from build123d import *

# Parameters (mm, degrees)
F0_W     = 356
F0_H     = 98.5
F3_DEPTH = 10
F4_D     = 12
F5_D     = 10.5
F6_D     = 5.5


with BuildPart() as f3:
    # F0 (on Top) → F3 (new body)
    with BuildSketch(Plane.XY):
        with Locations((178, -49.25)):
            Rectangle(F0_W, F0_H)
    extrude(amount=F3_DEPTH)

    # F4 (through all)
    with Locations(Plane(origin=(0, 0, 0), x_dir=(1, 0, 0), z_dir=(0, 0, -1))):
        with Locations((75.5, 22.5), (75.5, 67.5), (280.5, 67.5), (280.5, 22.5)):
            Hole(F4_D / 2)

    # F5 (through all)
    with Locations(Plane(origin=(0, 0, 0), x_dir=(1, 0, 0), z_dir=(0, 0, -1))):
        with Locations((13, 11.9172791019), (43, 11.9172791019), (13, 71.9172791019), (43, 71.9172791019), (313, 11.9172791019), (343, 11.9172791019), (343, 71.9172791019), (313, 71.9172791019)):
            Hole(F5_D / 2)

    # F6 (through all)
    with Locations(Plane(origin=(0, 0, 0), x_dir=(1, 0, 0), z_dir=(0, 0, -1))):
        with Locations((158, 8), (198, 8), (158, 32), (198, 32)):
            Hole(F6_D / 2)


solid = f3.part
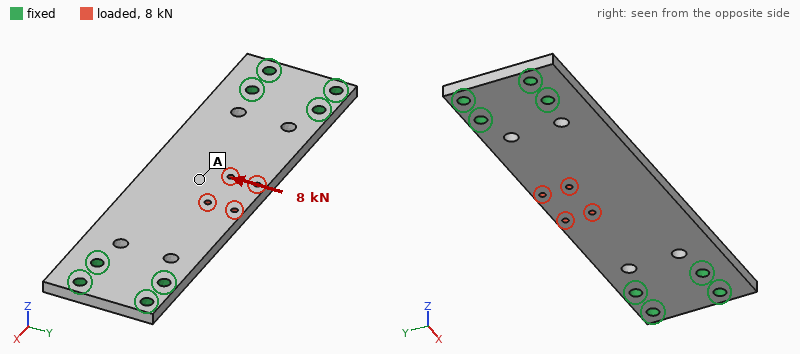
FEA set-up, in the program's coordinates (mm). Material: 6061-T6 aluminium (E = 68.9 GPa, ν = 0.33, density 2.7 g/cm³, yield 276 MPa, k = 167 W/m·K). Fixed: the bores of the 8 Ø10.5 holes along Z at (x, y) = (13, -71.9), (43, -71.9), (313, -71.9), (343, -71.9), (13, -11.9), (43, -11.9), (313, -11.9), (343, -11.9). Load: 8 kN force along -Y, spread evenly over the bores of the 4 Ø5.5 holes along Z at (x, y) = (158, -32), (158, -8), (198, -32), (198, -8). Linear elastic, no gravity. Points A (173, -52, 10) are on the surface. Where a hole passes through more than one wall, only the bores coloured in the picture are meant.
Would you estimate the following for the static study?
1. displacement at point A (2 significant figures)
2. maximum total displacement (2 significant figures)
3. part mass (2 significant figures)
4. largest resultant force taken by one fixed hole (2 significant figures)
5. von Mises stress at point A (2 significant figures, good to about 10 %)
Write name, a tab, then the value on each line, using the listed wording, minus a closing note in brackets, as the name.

displacement at point A	40 µm
maximum total displacement	42 µm
part mass	910 g
largest resultant force taken by one fixed hole	3.7 kN
von Mises stress at point A	4.8 MPa
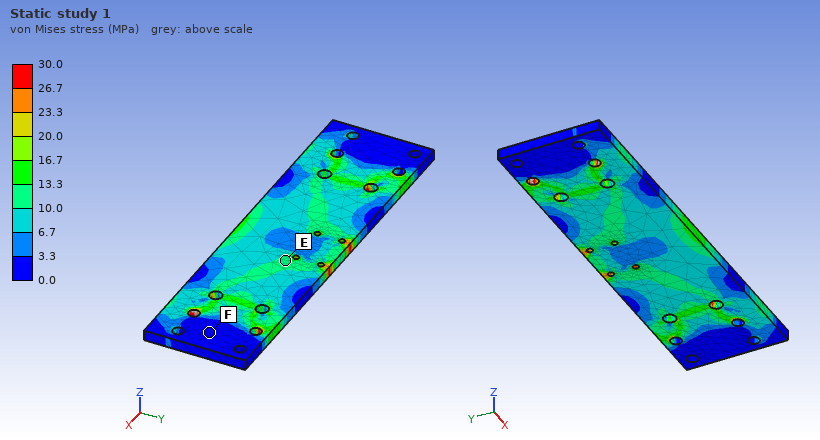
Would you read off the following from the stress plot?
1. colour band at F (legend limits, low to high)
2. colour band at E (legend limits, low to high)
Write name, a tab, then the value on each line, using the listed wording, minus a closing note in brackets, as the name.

colour band at F	0.0 to 3.3 MPa
colour band at E	10.0 to 13.3 MPa
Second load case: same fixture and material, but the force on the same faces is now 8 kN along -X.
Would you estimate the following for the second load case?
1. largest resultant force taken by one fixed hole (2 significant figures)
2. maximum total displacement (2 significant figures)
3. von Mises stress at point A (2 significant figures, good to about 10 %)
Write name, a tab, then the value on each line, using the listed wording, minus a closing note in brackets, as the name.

largest resultant force taken by one fixed hole	1.9 kN
maximum total displacement	13 µm
von Mises stress at point A	2.8 MPa
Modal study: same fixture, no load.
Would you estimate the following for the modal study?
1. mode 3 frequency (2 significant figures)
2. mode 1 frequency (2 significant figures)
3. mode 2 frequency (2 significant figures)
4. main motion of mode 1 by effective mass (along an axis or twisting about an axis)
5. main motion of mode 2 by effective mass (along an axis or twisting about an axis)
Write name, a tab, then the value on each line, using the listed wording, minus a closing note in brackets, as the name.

mode 3 frequency	2000 Hz
mode 1 frequency	710 Hz
mode 2 frequency	1400 Hz
main motion of mode 1 by effective mass	along Z
main motion of mode 2 by effective mass	twisting about X
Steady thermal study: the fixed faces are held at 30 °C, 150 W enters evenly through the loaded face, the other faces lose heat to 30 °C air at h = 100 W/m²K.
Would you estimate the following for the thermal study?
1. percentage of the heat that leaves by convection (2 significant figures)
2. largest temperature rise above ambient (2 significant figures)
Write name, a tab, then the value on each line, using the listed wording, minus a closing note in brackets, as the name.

percentage of the heat that leaves by convection	61 %
largest temperature rise above ambient	45 K
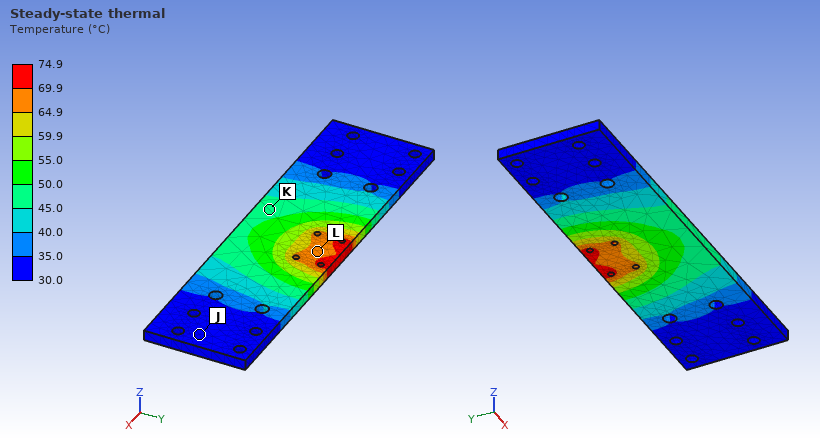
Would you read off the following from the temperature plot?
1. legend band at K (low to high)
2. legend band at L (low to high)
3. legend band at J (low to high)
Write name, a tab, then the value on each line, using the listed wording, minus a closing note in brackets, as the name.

legend band at K	45.0 to 50.0 °C
legend band at L	64.9 to 69.9 °C
legend band at J	30.0 to 35.0 °C
